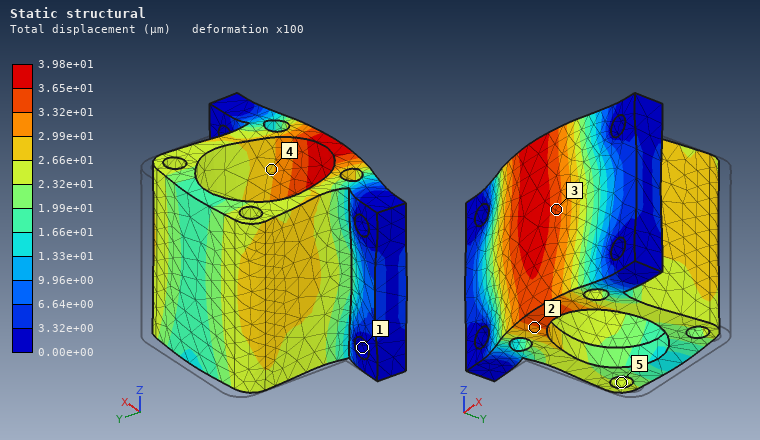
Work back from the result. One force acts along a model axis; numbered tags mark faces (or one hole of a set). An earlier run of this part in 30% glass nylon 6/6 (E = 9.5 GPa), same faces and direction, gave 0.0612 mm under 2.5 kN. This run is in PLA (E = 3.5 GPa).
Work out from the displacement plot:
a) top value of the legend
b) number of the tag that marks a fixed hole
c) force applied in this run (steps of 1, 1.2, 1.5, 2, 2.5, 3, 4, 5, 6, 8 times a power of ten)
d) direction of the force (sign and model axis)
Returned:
3.98e+01 µm
1
600 N
-Y
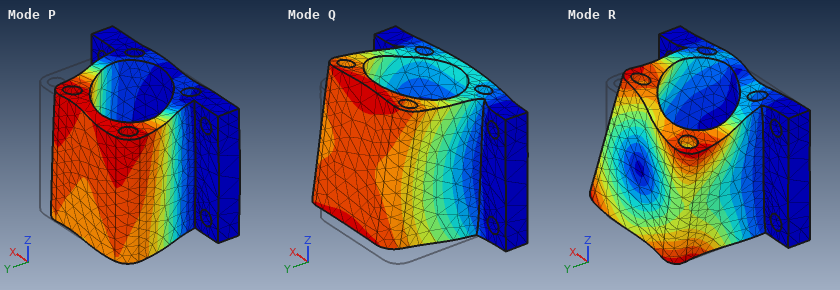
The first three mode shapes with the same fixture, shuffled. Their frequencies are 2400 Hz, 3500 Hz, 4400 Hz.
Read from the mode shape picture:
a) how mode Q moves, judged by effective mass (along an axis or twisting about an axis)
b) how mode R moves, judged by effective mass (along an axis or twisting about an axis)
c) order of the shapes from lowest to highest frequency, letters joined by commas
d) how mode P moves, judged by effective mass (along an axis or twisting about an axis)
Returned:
along Z
twisting about Y
P, Q, R
along X
